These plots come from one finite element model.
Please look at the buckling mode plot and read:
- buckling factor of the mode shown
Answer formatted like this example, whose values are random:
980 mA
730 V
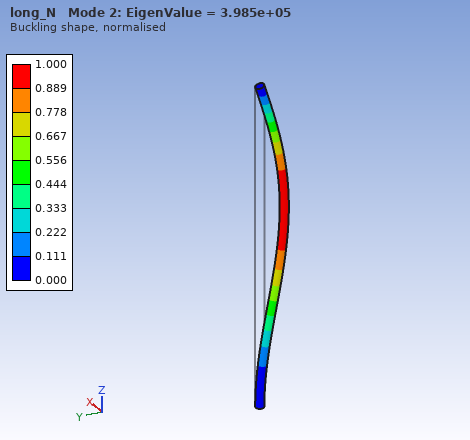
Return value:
3.985e+05
